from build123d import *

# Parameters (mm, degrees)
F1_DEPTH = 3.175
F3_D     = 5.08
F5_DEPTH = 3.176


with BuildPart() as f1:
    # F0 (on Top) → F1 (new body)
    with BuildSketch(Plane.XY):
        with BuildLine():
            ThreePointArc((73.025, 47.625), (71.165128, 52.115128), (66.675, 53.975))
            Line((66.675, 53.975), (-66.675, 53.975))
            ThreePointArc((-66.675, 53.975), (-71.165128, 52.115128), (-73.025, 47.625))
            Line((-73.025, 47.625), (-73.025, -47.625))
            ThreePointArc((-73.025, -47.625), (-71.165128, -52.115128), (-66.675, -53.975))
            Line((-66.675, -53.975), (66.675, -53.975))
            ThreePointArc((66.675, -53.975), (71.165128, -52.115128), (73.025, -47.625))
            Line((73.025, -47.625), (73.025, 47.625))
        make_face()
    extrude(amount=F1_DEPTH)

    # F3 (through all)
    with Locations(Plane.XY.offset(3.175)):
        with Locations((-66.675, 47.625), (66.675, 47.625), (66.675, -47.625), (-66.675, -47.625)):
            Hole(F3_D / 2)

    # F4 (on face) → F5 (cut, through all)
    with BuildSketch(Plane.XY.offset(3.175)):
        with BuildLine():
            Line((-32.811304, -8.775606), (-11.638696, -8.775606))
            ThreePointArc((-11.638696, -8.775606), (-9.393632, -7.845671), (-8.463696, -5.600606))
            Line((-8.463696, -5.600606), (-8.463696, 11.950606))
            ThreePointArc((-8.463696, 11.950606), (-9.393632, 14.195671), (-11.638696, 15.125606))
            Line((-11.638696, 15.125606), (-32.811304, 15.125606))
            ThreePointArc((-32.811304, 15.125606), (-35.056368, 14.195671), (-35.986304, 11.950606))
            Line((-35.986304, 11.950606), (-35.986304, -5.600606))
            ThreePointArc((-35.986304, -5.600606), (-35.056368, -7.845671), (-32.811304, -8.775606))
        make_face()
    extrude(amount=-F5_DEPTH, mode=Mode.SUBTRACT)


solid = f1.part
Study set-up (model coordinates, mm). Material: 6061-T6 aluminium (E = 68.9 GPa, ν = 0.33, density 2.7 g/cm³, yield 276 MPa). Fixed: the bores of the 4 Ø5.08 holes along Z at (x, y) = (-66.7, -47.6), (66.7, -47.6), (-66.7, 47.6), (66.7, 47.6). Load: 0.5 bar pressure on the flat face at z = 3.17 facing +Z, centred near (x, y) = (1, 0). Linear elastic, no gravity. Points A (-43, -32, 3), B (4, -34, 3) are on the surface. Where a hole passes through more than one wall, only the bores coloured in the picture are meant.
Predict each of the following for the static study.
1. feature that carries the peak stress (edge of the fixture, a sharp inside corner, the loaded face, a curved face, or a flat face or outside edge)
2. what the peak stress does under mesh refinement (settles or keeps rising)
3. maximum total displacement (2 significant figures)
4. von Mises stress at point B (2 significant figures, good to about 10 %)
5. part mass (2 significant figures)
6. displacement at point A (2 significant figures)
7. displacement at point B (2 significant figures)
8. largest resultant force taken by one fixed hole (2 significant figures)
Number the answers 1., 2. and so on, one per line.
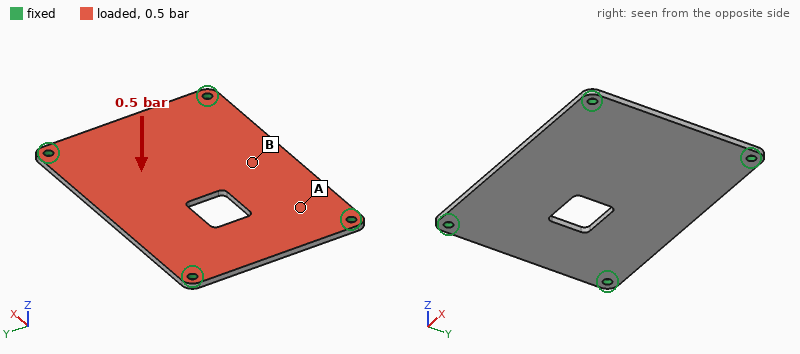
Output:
1. edge of the fixture
2. keeps rising
3. 0.42 mm
4. 26 MPa
5. 130 g
6. 0.17 mm
7. 0.35 mm
8. 190 N
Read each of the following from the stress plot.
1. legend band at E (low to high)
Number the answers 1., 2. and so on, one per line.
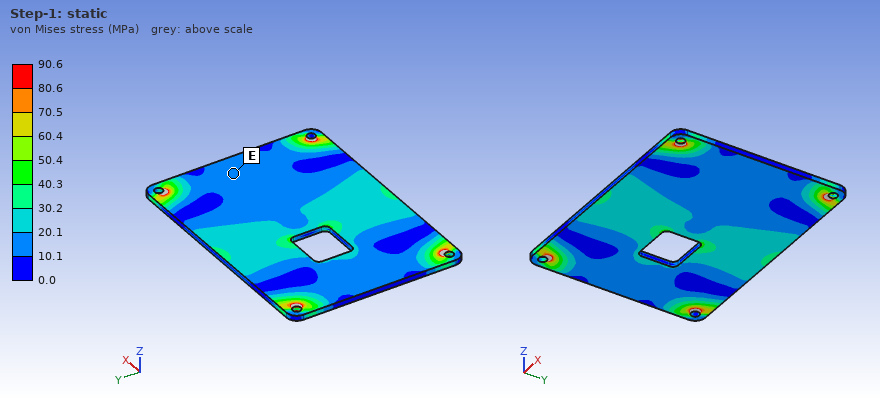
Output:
1. 10.1 to 20.1 MPa
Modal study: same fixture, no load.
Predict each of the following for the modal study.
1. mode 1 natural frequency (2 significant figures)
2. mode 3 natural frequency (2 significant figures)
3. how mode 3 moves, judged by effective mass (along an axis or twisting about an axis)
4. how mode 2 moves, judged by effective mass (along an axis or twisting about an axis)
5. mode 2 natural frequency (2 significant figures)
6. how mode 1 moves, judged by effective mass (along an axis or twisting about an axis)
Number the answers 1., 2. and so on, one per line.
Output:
1. 720 Hz
2. 1700 Hz
3. twisting about Y
4. twisting about X
5. 1200 Hz
6. along Z
